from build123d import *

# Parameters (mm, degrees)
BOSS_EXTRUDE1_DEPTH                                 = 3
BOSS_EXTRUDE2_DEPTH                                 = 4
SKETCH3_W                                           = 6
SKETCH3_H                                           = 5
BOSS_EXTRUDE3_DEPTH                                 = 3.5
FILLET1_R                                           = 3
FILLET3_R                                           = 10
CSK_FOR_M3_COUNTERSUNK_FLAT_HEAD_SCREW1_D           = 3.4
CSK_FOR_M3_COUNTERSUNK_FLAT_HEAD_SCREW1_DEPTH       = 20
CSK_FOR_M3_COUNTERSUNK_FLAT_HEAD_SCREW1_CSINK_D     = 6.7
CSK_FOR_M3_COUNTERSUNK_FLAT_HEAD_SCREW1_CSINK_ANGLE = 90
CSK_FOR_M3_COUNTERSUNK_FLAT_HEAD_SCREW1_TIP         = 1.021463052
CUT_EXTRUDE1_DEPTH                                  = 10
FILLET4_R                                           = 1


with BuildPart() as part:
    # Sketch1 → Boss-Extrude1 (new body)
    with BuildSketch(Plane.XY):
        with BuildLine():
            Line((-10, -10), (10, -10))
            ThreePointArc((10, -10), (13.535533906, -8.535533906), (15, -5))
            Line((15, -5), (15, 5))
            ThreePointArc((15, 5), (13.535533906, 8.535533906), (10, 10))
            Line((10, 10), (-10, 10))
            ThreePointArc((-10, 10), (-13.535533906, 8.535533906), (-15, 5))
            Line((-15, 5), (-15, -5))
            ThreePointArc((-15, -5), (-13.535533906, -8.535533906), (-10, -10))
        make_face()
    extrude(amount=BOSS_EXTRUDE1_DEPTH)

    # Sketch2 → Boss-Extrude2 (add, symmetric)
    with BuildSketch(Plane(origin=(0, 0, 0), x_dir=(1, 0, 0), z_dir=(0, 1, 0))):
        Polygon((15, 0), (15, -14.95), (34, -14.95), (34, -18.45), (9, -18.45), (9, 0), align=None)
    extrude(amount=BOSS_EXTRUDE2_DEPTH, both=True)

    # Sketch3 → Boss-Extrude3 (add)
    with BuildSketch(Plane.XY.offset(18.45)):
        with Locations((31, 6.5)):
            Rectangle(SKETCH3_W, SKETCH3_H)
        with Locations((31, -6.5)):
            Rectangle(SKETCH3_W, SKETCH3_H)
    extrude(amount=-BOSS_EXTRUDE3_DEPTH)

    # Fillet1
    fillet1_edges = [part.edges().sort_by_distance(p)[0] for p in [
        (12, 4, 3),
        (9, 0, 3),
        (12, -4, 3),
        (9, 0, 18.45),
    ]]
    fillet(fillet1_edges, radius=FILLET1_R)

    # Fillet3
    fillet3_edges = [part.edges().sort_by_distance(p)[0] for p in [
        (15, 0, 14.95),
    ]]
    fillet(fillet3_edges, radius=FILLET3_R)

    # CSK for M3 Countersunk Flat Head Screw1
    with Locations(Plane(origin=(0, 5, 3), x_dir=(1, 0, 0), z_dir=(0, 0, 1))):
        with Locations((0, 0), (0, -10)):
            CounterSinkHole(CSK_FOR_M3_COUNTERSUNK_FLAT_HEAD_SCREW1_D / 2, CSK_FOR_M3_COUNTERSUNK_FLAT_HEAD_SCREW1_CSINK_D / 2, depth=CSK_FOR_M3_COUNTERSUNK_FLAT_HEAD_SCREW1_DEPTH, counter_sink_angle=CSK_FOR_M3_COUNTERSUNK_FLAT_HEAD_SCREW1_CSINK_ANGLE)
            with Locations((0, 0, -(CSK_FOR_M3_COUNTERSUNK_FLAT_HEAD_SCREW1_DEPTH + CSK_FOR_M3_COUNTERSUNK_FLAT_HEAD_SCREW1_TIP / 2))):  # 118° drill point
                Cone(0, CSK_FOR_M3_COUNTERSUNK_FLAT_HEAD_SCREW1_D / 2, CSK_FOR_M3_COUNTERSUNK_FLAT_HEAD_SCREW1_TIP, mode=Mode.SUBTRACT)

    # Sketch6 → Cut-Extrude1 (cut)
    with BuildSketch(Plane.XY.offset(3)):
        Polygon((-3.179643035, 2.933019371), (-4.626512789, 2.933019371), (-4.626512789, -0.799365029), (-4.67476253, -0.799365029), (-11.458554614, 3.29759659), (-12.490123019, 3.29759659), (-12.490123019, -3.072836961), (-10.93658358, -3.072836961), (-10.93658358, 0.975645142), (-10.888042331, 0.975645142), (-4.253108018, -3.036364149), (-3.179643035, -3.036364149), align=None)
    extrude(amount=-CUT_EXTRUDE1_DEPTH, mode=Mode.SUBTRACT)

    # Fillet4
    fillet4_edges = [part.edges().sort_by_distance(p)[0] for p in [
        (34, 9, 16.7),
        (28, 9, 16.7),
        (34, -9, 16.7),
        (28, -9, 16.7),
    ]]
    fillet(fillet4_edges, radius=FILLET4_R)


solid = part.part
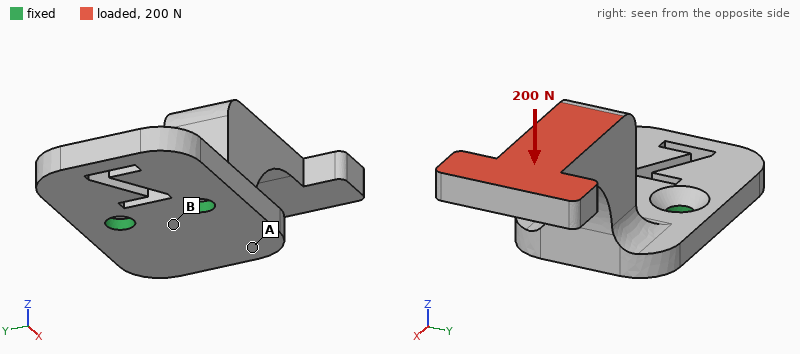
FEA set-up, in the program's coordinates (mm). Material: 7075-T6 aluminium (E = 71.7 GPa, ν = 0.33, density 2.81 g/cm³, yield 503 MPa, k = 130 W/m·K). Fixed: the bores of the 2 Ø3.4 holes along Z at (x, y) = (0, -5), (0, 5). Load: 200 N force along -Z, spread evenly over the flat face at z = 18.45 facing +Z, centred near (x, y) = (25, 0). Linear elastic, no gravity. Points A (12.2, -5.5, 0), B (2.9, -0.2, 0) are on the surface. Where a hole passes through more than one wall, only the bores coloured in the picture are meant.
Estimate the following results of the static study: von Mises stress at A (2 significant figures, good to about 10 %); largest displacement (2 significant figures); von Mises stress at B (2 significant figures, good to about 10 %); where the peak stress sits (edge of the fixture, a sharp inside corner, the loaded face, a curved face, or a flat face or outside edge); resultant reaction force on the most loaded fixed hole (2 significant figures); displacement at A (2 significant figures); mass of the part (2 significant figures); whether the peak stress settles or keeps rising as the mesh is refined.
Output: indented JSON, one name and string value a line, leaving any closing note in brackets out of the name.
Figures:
{
  "von Mises stress at A": "33 MPa",
  "largest displacement": "0.63 mm",
  "von Mises stress at B": "140 MPa",
  "where the peak stress sits": "edge of the fixture",
  "resultant reaction force on the most loaded fixed hole": "100 N",
  "displacement at A": "0.14 mm",
  "mass of the part": "9.1 g",
  "whether the peak stress settles or keeps rising as the mesh is refined": "keeps rising"
}
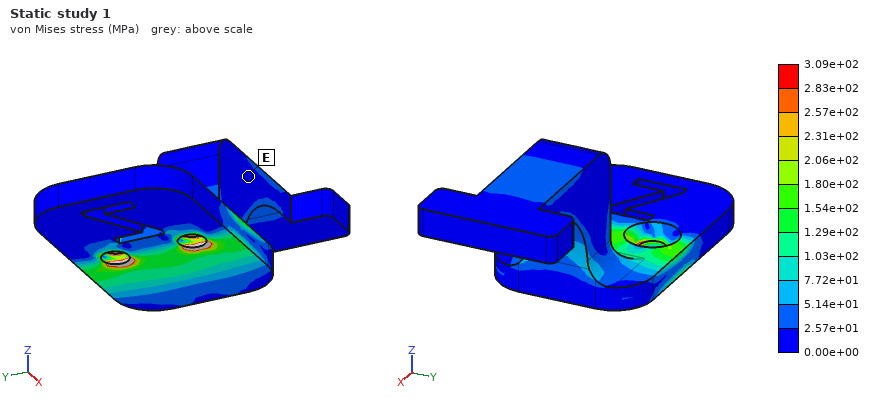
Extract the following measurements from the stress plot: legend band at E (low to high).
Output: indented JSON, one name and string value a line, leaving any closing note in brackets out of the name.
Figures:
{
  "legend band at E": "0.00e+00 to 2.57e+01 MPa"
}
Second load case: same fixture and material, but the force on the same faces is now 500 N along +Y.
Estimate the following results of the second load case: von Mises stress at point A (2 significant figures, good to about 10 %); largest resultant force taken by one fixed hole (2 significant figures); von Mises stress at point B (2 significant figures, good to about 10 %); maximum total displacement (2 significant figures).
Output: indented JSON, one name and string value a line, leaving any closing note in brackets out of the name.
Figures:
{
  "von Mises stress at point A": "68 MPa",
  "largest resultant force taken by one fixed hole": "1.4 kN",
  "von Mises stress at point B": "94 MPa",
  "maximum total displacement": "0.37 mm"
}
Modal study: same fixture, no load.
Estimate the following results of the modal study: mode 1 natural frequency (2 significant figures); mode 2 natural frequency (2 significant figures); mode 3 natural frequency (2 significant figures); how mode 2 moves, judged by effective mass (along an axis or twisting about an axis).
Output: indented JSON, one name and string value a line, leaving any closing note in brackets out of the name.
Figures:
{
  "mode 1 natural frequency": "1700 Hz",
  "mode 2 natural frequency": "4200 Hz",
  "mode 3 natural frequency": "8600 Hz",
  "how mode 2 moves, judged by effective mass": "along Y"
}
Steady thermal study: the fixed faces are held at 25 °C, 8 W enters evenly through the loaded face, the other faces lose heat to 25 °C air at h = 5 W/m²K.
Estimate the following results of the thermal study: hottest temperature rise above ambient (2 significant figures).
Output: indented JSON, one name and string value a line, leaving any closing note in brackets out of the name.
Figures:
{
  "hottest temperature rise above ambient": "43 K"
}
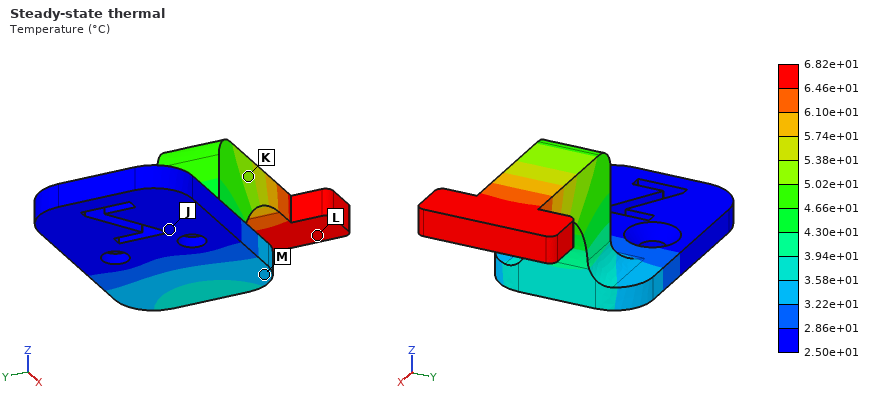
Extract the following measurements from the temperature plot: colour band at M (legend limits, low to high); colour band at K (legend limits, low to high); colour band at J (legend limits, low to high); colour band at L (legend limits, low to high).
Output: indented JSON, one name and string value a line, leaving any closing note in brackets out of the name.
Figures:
{
  "colour band at M": "3.22e+01 to 3.58e+01 °C",
  "colour band at K": "5.02e+01 to 5.38e+01 °C",
  "colour band at J": "2.50e+01 to 2.86e+01 °C",
  "colour band at L": "6.46e+01 to 6.82e+01 °C"
}
